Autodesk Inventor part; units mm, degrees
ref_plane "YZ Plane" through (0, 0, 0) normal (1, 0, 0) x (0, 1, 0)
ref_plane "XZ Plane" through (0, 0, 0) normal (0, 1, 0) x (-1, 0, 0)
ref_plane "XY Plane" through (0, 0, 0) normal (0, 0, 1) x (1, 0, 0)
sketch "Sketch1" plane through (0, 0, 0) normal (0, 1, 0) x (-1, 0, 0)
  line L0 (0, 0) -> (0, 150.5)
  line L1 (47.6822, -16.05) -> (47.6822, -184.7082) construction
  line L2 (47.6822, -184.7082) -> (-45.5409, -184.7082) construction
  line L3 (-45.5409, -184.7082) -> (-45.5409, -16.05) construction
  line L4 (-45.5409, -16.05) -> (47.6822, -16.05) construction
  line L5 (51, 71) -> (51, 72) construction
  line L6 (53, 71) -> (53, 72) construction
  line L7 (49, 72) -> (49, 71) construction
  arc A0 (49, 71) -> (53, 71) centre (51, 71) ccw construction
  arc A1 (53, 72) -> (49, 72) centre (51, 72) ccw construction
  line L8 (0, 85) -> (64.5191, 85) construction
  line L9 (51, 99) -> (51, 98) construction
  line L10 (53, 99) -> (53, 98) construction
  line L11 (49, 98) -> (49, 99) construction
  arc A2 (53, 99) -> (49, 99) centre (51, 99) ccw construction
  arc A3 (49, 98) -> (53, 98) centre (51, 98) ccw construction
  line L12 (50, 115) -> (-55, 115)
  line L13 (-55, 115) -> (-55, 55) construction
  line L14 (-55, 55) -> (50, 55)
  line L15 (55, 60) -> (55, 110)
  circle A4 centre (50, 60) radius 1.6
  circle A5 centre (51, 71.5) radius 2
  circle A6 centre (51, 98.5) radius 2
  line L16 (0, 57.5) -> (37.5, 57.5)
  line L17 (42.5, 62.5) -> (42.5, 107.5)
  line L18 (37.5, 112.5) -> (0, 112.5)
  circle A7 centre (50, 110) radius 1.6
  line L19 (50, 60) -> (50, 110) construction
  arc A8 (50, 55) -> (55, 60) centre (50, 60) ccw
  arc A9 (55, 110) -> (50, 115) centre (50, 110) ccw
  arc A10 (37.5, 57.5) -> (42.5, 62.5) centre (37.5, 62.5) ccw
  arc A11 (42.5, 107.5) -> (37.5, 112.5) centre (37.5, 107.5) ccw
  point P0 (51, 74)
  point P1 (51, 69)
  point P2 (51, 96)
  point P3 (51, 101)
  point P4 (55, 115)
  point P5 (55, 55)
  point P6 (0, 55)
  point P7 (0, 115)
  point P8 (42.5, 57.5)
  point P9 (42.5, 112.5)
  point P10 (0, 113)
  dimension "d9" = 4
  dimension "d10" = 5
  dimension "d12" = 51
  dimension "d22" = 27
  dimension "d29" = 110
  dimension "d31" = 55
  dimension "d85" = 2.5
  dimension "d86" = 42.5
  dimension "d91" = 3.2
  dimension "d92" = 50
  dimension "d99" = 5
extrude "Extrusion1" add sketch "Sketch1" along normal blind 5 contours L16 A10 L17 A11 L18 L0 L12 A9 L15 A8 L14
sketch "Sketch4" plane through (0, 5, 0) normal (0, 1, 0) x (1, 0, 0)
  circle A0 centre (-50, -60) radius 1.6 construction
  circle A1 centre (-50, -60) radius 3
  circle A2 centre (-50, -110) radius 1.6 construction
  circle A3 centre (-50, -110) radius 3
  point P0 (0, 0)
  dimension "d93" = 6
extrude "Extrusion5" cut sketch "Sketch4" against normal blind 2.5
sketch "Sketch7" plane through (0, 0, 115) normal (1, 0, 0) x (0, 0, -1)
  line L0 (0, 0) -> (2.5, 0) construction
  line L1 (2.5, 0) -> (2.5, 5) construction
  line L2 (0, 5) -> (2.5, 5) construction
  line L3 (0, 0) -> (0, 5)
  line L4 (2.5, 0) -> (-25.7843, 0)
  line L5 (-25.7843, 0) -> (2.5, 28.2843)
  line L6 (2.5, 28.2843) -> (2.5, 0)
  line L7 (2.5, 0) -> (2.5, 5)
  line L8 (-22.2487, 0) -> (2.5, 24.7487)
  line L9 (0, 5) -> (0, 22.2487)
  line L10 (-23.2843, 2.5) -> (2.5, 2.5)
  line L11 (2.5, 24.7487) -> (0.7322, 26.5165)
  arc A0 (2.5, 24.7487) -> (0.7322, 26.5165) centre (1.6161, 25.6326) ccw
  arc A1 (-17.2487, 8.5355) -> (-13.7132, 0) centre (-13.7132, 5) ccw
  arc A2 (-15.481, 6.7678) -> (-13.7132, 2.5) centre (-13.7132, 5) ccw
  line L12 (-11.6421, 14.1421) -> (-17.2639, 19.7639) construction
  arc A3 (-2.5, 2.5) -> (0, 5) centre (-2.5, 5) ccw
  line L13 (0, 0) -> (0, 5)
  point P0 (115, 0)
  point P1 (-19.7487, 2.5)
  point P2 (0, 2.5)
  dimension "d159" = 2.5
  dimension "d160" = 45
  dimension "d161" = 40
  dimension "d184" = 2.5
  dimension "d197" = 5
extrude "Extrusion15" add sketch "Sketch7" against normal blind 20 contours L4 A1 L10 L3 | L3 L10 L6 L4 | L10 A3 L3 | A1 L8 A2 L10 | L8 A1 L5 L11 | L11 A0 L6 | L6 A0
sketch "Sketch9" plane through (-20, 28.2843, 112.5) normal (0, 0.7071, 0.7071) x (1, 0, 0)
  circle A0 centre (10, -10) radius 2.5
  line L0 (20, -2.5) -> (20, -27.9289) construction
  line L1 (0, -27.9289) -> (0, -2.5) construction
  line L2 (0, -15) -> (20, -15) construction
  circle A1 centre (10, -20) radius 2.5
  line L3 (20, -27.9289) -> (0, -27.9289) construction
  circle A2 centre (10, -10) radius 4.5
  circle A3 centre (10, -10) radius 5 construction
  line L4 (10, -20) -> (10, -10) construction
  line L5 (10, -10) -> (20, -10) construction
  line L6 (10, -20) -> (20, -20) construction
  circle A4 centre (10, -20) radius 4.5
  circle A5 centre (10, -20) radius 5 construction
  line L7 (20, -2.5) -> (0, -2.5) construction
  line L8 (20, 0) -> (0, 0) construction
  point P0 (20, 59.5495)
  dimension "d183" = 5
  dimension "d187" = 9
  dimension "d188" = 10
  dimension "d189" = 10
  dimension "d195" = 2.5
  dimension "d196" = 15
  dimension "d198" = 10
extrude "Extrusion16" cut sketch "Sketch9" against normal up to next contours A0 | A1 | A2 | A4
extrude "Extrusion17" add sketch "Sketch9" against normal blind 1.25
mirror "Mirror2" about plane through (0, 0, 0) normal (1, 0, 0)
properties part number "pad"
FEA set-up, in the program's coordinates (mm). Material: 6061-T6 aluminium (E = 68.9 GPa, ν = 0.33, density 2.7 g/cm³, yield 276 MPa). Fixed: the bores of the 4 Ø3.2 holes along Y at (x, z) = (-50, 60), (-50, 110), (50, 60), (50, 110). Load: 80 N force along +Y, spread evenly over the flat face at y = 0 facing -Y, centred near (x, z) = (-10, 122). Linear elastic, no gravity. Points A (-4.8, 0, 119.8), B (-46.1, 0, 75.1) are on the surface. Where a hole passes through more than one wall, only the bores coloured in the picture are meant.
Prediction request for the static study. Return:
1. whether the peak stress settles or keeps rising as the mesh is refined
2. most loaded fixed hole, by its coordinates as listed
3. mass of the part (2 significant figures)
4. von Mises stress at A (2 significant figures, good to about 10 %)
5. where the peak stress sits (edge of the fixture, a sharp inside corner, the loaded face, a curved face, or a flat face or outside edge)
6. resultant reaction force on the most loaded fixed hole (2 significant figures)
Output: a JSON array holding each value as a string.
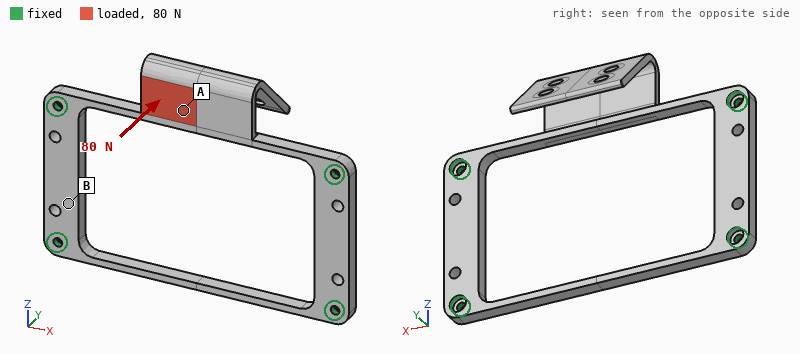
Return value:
["keeps rising", "(-50, 110)", "37 g", "16 MPa", "edge of the fixture", "64 N"]
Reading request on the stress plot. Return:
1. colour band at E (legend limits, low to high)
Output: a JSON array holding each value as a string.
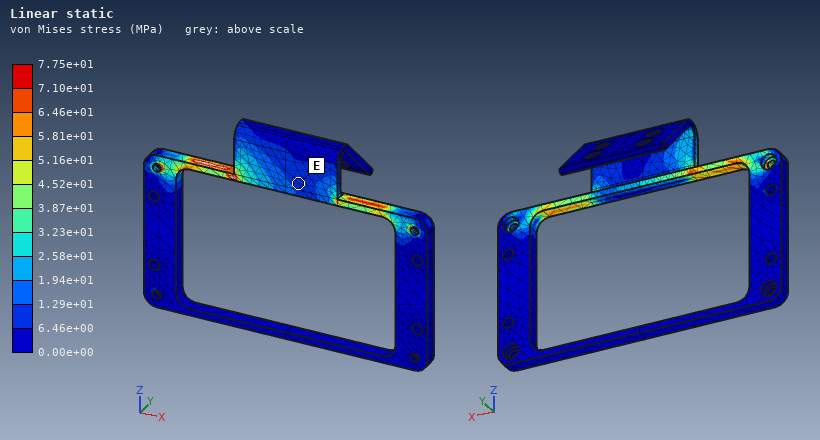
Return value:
["6.46e+00 to 1.29e+01 MPa"]
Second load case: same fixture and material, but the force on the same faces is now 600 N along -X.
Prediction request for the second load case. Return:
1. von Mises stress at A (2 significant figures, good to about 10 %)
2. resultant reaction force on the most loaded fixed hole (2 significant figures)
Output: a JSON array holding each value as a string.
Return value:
["9.4 MPa", "300 N"]
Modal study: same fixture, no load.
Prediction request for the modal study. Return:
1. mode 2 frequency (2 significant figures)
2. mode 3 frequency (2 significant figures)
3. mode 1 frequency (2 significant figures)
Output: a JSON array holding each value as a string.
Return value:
["1100 Hz", "1600 Hz", "530 Hz"]
